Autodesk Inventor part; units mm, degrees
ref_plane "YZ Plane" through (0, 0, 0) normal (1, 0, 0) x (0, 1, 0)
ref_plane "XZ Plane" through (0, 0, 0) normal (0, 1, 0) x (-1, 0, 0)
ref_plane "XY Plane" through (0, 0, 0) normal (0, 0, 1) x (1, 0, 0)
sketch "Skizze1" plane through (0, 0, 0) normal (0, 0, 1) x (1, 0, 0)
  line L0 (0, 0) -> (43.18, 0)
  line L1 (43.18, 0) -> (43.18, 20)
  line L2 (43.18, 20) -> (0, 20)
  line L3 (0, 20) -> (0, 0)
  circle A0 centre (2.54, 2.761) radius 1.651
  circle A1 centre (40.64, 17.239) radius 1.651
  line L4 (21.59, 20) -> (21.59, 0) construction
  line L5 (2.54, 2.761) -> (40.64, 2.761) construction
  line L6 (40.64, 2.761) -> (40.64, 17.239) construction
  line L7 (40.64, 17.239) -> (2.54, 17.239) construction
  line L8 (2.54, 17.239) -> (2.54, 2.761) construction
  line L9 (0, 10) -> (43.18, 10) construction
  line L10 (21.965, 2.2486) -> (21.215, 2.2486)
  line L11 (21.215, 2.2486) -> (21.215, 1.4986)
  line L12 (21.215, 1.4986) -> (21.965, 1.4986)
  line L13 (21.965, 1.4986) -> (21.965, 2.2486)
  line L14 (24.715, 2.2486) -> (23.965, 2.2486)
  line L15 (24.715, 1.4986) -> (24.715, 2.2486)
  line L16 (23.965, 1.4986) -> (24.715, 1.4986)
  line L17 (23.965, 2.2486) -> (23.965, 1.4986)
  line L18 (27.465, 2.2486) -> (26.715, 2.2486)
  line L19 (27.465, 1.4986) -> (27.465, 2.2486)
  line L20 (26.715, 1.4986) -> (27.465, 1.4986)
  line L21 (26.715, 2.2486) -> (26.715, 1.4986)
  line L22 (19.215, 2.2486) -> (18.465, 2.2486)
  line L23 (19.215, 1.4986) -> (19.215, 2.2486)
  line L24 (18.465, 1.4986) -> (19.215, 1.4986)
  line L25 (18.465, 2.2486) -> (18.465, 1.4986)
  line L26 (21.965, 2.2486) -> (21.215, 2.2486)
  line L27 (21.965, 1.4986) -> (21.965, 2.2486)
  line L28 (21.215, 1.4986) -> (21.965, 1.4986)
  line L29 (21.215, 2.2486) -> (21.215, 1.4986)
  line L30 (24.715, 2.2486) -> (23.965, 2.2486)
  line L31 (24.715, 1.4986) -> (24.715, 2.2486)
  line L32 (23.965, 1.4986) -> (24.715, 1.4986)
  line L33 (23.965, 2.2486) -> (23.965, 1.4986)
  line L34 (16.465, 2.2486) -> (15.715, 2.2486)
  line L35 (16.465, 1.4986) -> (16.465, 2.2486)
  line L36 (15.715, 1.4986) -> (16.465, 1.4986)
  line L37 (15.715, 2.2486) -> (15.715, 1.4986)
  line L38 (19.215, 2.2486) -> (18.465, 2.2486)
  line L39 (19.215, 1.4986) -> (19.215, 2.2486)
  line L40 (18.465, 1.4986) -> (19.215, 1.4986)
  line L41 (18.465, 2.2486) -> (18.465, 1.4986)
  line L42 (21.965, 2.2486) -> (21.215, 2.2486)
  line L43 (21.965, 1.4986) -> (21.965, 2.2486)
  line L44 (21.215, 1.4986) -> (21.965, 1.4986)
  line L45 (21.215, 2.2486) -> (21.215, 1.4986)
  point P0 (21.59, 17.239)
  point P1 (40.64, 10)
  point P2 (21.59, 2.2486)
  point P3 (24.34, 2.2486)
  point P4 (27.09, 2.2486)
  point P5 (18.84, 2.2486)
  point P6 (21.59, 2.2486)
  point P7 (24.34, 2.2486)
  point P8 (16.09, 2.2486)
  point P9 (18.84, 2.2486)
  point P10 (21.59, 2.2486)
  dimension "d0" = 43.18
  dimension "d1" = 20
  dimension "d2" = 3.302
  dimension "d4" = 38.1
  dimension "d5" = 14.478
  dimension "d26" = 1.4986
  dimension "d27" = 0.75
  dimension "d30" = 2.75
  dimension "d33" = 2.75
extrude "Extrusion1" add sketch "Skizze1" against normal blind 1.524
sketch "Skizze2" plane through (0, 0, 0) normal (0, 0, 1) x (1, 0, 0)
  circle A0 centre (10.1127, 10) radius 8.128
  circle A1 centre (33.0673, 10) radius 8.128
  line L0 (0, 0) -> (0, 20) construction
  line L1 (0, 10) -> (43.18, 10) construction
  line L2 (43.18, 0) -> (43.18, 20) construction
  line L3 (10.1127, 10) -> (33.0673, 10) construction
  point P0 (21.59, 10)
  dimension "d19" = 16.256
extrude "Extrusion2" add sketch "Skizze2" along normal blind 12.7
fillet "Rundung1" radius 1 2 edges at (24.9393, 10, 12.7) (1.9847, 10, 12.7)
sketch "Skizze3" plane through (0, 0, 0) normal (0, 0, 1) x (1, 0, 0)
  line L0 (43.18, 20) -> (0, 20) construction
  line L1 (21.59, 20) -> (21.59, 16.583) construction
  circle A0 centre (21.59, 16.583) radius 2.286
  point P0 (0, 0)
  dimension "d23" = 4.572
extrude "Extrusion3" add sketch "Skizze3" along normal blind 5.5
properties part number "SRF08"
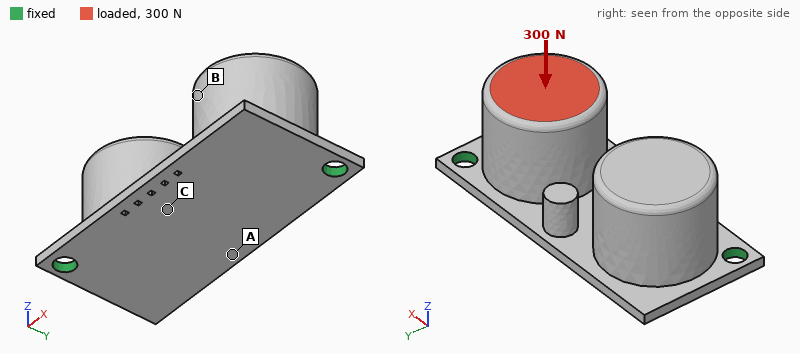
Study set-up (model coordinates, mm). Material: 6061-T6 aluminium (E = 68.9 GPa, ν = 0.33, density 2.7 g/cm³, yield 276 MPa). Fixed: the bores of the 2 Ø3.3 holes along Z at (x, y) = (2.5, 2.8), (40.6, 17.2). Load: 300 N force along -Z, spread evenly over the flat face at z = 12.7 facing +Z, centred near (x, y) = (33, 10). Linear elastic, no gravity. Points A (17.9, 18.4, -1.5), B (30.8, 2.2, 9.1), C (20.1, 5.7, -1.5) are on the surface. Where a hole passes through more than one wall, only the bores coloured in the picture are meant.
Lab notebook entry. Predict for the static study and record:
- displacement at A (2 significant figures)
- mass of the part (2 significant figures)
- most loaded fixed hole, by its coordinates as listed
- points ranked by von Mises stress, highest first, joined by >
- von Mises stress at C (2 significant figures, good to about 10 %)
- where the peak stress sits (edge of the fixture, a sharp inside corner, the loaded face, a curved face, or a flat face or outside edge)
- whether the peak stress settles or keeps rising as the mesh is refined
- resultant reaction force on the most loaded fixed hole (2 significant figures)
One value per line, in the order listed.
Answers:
0.062 mm
18 g
(40.6, 17.2)
A > C > B
33 MPa
edge of the fixture
keeps rising
230 N
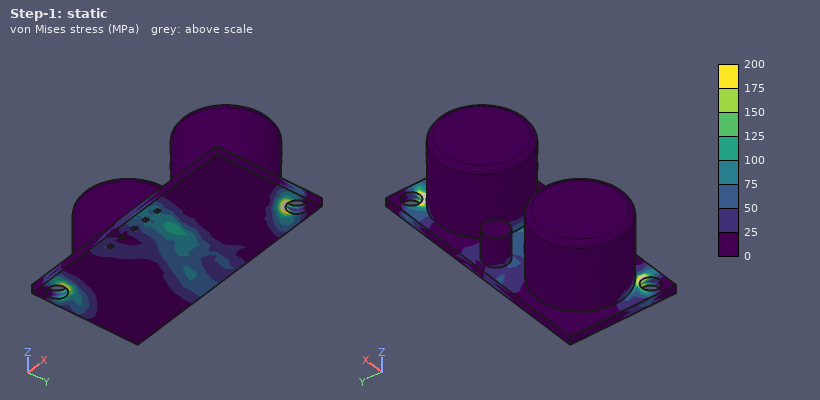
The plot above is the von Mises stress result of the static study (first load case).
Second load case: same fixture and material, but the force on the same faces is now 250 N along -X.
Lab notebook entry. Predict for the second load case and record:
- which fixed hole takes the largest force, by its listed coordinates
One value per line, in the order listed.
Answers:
(40.6, 17.2)
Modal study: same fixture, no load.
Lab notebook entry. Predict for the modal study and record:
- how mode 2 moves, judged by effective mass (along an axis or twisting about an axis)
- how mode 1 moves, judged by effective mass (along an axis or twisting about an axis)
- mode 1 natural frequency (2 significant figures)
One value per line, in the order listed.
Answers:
along Y
along Z
2100 Hz
